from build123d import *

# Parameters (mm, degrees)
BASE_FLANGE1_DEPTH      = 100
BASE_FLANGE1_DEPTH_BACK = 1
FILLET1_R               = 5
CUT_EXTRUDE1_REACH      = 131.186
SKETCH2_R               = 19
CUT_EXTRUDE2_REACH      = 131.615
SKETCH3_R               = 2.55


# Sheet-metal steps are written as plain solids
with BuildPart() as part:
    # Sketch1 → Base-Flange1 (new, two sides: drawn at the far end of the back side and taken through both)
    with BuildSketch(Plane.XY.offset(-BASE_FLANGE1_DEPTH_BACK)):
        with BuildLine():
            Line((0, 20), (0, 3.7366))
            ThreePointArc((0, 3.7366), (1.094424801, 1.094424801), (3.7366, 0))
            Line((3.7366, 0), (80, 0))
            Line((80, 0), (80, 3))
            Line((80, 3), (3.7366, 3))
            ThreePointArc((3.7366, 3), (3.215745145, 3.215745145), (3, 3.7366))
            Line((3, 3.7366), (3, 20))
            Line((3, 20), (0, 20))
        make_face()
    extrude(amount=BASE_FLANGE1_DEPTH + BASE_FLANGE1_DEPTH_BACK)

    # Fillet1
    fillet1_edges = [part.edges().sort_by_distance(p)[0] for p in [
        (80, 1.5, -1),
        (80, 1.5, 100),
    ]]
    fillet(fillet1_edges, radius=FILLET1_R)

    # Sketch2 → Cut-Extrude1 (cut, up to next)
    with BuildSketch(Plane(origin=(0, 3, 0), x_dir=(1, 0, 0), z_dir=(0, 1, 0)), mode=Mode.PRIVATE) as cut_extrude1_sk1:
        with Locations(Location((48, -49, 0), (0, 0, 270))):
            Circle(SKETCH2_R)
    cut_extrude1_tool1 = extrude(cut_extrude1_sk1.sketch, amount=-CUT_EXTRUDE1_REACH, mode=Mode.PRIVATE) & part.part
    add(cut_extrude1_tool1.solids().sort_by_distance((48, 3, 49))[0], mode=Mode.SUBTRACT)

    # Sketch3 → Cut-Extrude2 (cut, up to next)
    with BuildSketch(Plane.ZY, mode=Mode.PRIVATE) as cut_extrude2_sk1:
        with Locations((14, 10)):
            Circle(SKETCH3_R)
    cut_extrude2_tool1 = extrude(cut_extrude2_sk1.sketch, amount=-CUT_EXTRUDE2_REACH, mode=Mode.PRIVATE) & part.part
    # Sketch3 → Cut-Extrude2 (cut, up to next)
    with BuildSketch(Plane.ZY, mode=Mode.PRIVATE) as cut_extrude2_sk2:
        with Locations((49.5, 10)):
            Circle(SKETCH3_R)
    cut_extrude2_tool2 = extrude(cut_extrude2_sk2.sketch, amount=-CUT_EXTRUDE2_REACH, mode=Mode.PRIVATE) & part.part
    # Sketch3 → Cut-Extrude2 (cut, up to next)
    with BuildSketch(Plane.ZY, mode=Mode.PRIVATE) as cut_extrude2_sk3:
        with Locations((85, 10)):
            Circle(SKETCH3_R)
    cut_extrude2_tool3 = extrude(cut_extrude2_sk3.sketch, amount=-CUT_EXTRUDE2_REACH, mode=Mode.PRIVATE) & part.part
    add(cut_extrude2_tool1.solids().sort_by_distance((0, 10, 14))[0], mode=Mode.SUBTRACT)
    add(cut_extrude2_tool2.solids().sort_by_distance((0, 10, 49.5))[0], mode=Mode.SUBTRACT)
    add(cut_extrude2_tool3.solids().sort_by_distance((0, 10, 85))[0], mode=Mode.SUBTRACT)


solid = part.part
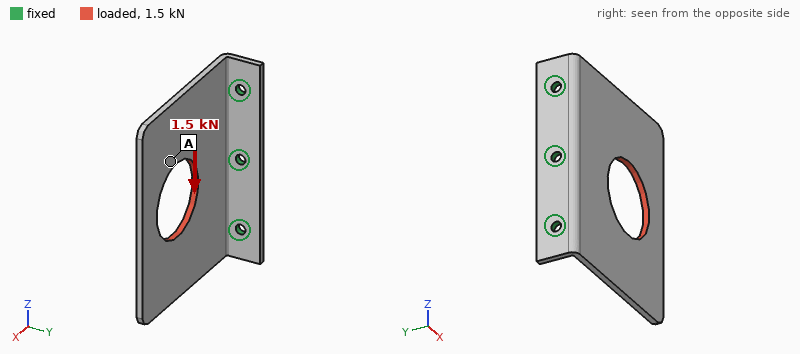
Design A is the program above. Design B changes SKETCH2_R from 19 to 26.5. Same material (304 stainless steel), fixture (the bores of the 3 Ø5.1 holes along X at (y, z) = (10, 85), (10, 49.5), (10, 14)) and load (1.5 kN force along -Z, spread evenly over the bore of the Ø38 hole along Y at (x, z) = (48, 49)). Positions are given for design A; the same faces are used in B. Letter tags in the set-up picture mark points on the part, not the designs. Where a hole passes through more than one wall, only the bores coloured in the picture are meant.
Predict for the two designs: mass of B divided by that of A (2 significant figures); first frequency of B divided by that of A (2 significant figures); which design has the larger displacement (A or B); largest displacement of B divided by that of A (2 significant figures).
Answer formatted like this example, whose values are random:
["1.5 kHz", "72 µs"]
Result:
["0.87", "1.0", "B", "1.2"]
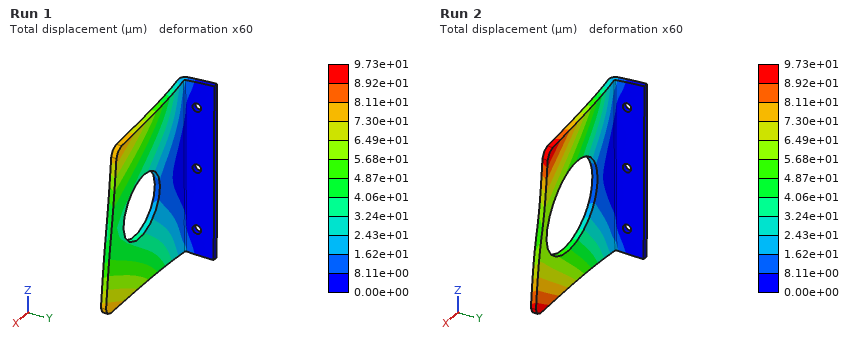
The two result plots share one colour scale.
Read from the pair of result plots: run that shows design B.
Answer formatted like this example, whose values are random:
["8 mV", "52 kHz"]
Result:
["Run 2"]
